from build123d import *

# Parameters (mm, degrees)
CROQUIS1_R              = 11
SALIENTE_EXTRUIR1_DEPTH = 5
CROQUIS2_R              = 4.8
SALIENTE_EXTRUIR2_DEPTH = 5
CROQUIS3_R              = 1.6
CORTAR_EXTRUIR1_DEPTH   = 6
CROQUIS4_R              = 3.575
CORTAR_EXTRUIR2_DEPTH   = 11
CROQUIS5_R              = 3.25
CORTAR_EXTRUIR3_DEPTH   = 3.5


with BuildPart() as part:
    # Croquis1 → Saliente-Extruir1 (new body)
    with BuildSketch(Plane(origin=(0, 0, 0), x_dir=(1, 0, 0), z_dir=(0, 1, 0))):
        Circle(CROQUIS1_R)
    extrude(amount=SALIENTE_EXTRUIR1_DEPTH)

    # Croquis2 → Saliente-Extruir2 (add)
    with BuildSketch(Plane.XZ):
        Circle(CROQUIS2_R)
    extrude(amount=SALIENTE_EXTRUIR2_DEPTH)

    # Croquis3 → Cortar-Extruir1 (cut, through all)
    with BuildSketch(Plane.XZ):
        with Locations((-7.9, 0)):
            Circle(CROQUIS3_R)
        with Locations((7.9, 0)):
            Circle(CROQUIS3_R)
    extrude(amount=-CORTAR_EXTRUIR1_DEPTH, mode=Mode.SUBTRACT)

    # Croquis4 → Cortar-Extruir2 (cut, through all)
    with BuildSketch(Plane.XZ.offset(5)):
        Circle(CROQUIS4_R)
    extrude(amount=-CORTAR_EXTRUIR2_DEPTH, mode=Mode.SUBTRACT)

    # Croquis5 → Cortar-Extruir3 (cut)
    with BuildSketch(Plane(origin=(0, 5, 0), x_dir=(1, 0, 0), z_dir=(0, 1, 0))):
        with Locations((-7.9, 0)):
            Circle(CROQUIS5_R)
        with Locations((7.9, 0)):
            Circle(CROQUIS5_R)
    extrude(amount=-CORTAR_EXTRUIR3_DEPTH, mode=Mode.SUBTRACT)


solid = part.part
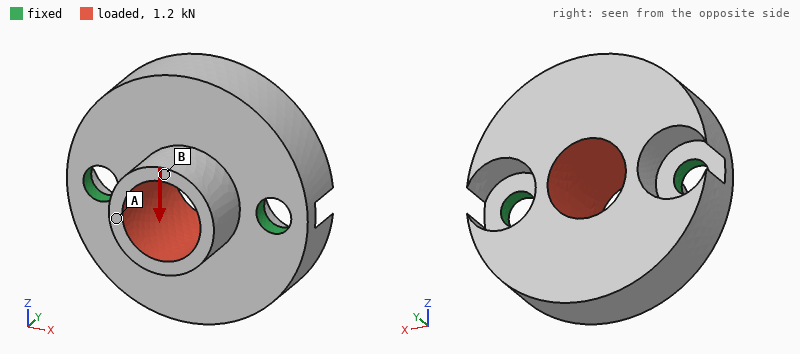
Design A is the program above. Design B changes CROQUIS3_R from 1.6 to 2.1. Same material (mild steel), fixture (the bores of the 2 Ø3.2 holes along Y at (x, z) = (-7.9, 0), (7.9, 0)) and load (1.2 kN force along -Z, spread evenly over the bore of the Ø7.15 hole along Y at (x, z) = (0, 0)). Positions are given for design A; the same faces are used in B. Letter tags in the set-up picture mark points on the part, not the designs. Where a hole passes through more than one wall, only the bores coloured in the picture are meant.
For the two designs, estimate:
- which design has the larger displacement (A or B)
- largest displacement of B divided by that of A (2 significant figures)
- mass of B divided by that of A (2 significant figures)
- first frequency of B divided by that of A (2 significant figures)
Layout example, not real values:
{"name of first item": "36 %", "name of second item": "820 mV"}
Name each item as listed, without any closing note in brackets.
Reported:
{"which design has the larger displacement": "A", "largest displacement of B divided by that of A": "0.79", "mass of B divided by that of A": "0.99", "first frequency of B divided by that of A": "1.3"}
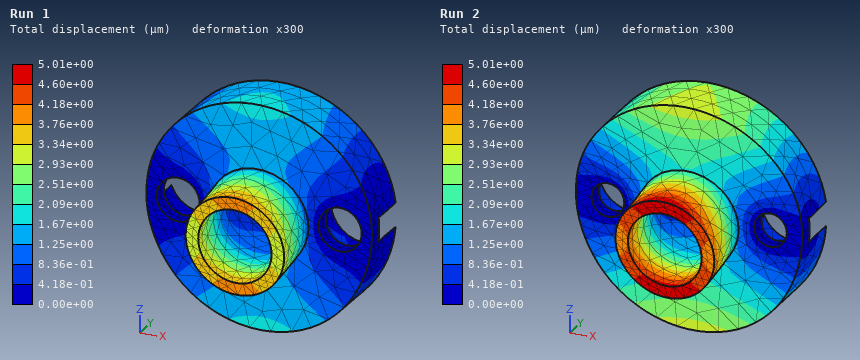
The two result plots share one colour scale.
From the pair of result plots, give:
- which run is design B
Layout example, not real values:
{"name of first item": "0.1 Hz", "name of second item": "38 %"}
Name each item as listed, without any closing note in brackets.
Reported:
{"which run is design B": "Run 1"}
